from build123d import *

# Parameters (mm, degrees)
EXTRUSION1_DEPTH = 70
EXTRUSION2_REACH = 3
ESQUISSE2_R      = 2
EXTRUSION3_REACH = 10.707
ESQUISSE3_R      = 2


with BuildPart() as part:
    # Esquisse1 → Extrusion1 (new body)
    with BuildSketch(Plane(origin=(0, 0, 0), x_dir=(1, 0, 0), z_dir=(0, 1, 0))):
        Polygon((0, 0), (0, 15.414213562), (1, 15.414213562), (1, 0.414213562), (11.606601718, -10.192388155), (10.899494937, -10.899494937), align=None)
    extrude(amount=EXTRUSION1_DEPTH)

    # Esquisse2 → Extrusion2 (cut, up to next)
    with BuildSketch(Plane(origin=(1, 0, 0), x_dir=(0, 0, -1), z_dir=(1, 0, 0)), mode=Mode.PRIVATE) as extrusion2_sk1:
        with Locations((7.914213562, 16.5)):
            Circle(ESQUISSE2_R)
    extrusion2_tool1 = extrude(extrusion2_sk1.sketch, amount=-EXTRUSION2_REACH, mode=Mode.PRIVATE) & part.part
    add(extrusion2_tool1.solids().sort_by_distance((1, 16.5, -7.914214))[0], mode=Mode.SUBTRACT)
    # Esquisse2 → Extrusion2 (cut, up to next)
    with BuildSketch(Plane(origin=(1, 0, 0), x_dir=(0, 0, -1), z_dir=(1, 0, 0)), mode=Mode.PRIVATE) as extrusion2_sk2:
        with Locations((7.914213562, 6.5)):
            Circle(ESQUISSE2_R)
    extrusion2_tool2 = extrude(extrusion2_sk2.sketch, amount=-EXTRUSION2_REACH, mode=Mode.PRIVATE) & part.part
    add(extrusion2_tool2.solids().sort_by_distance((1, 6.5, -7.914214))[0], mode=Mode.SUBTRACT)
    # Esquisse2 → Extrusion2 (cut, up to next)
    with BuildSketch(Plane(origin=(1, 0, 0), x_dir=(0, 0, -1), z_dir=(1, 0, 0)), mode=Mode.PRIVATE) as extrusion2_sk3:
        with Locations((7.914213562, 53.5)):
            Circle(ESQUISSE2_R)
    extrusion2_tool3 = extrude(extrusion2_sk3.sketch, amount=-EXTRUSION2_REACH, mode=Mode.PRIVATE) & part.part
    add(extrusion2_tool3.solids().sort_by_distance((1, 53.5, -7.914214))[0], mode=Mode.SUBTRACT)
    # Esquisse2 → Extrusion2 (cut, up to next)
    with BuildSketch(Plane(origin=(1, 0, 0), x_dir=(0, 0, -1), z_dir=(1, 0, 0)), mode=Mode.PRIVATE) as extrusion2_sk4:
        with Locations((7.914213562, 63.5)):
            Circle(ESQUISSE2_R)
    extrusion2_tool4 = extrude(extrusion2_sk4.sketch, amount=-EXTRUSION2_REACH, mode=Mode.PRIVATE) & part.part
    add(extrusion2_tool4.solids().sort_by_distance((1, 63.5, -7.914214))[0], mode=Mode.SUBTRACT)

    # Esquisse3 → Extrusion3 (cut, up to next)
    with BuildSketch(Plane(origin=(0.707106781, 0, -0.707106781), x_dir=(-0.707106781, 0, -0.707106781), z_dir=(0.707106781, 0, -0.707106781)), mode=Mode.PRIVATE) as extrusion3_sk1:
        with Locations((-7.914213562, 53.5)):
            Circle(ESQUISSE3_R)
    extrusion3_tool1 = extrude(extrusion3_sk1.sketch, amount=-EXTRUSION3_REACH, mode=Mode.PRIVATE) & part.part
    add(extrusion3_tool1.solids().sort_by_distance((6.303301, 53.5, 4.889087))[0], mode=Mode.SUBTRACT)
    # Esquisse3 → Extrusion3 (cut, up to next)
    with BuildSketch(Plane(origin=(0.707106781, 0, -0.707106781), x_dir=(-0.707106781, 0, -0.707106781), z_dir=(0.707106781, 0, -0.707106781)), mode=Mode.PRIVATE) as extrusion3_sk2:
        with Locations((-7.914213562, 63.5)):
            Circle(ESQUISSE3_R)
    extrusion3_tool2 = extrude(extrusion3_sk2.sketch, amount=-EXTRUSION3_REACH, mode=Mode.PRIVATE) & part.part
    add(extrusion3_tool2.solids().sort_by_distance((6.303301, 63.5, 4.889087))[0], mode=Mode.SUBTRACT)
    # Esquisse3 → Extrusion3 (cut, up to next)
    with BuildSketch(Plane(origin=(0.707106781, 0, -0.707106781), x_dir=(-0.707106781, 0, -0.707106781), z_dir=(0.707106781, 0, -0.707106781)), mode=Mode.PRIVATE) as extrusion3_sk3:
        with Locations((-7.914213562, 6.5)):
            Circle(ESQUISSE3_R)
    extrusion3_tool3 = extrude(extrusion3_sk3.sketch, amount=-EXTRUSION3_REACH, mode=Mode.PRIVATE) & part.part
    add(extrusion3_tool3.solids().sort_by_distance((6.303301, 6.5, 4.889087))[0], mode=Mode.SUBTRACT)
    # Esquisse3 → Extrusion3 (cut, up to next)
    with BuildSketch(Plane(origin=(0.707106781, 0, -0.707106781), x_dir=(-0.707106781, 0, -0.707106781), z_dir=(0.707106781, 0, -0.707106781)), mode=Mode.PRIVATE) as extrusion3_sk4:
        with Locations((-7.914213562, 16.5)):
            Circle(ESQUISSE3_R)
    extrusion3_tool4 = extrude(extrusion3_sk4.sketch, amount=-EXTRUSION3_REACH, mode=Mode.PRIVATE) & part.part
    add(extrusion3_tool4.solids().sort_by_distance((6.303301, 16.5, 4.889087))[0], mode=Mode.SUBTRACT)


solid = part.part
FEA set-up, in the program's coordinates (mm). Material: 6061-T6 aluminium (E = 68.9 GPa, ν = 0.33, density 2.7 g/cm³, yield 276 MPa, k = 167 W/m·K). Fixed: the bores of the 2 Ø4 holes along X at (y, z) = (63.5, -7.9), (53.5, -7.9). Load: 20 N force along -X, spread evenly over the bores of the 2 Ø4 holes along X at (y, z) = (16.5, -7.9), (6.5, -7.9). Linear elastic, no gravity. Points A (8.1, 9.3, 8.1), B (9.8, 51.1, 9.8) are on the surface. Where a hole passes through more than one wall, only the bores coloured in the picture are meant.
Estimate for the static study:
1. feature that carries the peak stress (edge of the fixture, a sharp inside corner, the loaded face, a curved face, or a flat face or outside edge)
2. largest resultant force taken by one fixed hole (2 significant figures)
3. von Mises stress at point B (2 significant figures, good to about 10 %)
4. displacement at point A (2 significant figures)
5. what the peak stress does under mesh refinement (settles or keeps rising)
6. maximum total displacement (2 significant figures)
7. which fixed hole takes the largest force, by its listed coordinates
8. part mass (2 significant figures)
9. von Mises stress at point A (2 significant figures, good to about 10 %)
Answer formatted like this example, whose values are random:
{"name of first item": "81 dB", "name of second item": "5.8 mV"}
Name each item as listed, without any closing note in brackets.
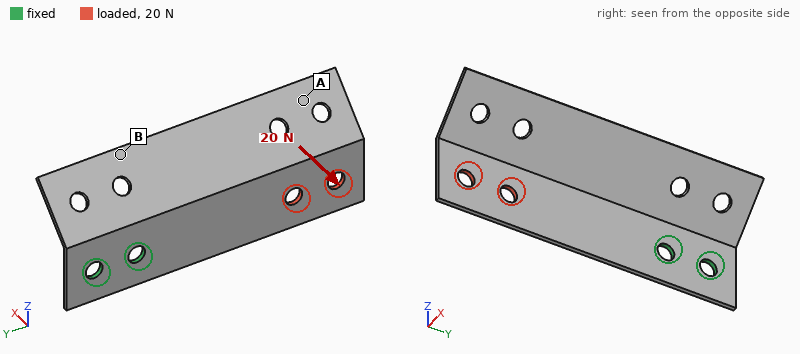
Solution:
{"feature that carries the peak stress": "edge of the fixture", "largest resultant force taken by one fixed hole": "72 N", "von Mises stress at point B": "31 MPa", "displacement at point A": "0.28 mm", "what the peak stress does under mesh refinement": "keeps rising", "maximum total displacement": "0.74 mm", "which fixed hole takes the largest force, by its listed coordinates": "(53.5, -7.9)", "part mass": "5.5 g", "von Mises stress at point A": "9.5 MPa"}
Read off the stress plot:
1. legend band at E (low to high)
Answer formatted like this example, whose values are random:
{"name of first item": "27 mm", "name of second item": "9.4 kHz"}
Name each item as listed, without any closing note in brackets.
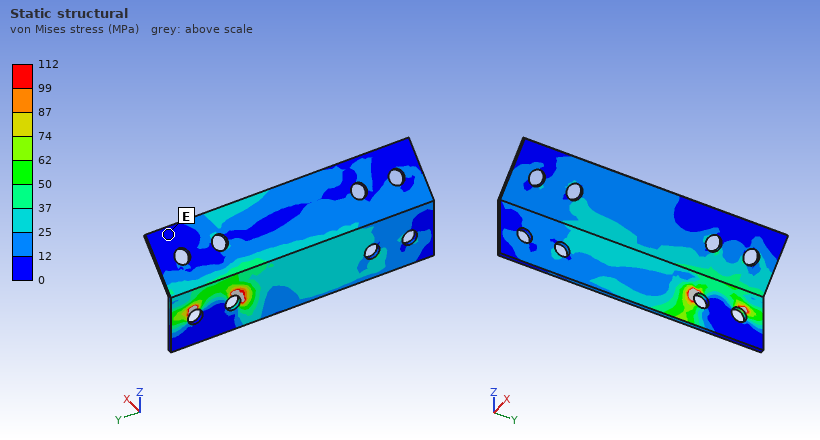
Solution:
{"legend band at E": "0 to 12 MPa"}
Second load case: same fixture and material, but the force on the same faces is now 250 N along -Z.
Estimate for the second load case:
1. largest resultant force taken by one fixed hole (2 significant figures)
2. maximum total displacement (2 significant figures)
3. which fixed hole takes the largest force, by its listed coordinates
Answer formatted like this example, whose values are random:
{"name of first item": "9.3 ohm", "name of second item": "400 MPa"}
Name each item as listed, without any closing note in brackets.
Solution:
{"largest resultant force taken by one fixed hole": "860 N", "maximum total displacement": "0.74 mm", "which fixed hole takes the largest force, by its listed coordinates": "(53.5, -7.9)"}
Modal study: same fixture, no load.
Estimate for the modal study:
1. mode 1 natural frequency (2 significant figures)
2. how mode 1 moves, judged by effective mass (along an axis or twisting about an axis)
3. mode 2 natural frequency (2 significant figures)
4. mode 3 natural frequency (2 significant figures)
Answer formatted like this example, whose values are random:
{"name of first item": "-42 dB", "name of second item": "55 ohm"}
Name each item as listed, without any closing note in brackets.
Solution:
{"mode 1 natural frequency": "680 Hz", "how mode 1 moves, judged by effective mass": "along X", "mode 2 natural frequency": "1000 Hz", "mode 3 natural frequency": "2100 Hz"}
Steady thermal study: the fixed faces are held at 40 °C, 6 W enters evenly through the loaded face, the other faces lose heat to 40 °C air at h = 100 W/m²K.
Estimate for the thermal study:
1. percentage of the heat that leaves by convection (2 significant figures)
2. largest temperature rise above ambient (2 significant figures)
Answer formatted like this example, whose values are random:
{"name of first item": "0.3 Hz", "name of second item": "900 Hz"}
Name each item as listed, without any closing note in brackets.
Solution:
{"percentage of the heat that leaves by convection": "73 %", "largest temperature rise above ambient": "30 K"}
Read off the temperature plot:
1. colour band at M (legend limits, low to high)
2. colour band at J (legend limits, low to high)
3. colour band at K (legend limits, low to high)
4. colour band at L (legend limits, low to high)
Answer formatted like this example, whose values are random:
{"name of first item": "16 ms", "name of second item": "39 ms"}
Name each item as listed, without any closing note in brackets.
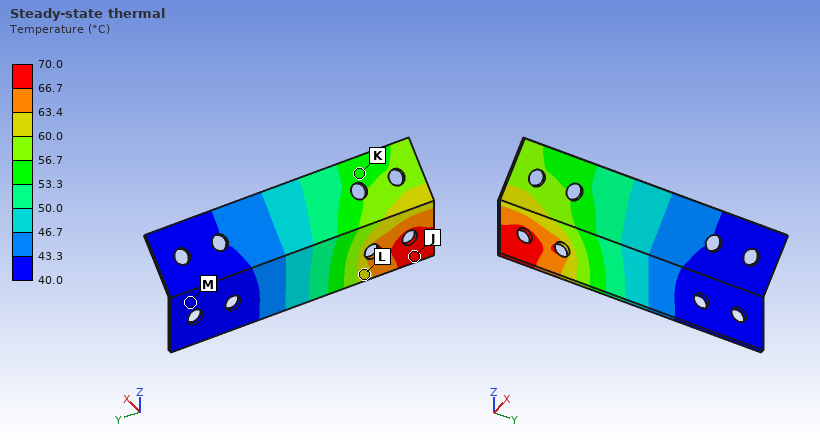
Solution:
{"colour band at M": "40.0 to 43.3 °C", "colour band at J": "66.7 to 70.0 °C", "colour band at K": "53.3 to 56.7 °C", "colour band at L": "60.0 to 63.4 °C"}
